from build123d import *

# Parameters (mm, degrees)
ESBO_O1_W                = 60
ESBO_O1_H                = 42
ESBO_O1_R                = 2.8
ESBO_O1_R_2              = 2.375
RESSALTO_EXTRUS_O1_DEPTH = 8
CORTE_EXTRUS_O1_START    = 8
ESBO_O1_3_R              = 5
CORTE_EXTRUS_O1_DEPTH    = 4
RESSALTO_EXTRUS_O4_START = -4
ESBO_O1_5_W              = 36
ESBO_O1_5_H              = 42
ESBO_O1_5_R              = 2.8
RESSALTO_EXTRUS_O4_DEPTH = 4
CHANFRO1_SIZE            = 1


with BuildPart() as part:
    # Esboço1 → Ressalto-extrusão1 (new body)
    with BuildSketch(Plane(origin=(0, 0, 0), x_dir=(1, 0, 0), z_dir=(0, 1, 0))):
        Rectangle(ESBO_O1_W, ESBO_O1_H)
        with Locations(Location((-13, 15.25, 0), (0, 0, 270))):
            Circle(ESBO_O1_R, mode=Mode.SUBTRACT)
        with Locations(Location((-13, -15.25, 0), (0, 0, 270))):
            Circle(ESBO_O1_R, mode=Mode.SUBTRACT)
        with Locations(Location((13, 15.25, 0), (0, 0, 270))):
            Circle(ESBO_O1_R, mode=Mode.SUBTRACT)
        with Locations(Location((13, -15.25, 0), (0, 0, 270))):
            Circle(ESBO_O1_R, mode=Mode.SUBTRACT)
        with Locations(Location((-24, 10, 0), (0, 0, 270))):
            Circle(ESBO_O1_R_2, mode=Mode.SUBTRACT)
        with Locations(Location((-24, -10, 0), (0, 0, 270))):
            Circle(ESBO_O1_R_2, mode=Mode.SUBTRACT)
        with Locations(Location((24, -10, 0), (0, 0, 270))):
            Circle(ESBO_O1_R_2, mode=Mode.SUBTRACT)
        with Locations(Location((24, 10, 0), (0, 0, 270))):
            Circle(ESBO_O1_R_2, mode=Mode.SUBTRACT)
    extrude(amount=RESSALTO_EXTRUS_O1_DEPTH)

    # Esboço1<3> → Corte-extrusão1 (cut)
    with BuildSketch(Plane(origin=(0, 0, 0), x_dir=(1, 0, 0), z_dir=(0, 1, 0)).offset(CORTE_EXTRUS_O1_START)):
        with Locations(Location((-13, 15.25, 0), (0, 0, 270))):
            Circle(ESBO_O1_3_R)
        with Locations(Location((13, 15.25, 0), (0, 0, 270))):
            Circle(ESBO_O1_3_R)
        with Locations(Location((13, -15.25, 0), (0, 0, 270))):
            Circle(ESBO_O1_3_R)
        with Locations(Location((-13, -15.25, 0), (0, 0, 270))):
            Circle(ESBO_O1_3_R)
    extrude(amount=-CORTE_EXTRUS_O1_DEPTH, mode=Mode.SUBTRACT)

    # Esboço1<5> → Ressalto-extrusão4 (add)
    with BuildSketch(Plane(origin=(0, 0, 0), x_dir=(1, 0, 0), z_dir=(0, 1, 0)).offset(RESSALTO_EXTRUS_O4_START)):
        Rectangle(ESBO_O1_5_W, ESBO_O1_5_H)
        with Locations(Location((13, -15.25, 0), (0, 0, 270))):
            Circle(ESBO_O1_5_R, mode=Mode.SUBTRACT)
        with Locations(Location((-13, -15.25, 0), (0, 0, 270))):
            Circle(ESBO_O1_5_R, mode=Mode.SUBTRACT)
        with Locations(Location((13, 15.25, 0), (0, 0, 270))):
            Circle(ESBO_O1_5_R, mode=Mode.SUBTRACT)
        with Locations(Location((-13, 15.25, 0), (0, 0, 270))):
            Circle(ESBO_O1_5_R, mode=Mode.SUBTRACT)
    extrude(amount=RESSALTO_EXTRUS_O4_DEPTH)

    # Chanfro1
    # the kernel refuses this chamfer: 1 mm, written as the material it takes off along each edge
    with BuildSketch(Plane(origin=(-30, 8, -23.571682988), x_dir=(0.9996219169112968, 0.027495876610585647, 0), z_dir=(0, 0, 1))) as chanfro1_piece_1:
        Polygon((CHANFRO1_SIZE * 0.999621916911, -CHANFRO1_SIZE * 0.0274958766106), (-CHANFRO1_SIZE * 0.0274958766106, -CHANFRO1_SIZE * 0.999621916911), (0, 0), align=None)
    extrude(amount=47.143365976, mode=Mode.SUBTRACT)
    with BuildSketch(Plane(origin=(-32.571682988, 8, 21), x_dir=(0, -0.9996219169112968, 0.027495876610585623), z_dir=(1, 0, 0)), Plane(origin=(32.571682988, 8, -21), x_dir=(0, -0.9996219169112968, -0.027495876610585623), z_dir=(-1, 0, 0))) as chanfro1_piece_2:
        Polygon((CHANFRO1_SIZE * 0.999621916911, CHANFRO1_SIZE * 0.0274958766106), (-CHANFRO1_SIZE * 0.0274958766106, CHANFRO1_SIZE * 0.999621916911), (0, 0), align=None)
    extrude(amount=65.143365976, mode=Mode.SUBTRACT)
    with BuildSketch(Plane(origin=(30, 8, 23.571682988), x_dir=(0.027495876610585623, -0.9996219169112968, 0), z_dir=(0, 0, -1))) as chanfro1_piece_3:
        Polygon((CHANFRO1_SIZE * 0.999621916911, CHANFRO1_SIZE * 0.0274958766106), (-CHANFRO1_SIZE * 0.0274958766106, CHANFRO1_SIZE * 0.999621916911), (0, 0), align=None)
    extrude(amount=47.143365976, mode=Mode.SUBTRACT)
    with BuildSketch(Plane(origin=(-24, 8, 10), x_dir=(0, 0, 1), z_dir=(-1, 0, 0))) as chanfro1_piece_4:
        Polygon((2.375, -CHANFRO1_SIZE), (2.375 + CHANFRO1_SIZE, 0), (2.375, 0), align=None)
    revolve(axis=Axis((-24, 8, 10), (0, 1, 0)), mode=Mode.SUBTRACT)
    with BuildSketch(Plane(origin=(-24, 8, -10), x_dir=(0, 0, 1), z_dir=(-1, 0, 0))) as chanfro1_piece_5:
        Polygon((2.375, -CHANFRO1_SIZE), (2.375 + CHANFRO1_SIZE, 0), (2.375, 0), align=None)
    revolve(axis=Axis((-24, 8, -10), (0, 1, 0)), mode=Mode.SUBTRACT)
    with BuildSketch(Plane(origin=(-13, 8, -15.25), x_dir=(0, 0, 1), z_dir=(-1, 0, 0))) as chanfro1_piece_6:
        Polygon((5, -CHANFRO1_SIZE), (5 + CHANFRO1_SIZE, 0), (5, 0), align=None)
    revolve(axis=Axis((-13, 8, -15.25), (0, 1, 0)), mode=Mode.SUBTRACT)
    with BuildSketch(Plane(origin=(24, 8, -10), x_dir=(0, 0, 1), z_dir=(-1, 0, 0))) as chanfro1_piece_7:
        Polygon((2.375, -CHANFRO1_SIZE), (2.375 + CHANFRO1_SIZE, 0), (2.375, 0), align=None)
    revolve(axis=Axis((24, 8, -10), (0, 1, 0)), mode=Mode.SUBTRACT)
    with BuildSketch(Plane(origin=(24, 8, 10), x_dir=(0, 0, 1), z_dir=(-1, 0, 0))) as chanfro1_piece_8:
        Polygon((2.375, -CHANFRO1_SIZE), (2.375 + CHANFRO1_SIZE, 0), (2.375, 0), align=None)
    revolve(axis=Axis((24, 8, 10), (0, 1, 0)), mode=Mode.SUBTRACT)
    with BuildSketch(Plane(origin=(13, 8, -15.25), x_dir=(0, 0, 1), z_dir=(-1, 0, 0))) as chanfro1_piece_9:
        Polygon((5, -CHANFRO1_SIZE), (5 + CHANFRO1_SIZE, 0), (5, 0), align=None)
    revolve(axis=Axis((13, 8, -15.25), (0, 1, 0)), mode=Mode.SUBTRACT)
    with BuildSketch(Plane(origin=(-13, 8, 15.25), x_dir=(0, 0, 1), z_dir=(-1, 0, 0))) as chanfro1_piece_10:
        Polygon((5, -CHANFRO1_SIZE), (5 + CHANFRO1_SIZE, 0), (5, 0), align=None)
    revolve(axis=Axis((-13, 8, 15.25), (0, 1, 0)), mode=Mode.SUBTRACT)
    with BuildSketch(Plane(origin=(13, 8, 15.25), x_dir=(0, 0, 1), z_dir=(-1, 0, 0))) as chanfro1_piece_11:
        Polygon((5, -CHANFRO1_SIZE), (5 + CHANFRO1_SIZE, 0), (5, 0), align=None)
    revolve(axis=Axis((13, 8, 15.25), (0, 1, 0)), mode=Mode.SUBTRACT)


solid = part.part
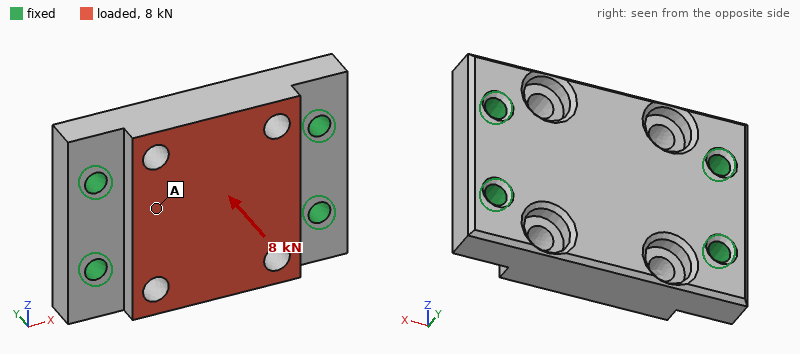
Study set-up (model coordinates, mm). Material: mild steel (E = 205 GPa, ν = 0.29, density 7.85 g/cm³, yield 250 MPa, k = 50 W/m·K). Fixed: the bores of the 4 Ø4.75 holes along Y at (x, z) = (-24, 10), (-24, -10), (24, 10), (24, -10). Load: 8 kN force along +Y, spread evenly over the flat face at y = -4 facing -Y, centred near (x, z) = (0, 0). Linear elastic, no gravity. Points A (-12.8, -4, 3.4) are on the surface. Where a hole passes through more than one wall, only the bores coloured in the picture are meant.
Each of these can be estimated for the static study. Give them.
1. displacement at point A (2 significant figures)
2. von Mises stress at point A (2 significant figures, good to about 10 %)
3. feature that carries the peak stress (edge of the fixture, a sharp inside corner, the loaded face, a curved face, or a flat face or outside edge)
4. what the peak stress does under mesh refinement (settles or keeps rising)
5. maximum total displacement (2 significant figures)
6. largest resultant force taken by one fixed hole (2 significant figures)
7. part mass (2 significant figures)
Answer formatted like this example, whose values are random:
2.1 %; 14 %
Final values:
5.3 µm; 16 MPa; edge of the fixture; keeps rising; 9.4 µm; 2.2 kN; 180 g
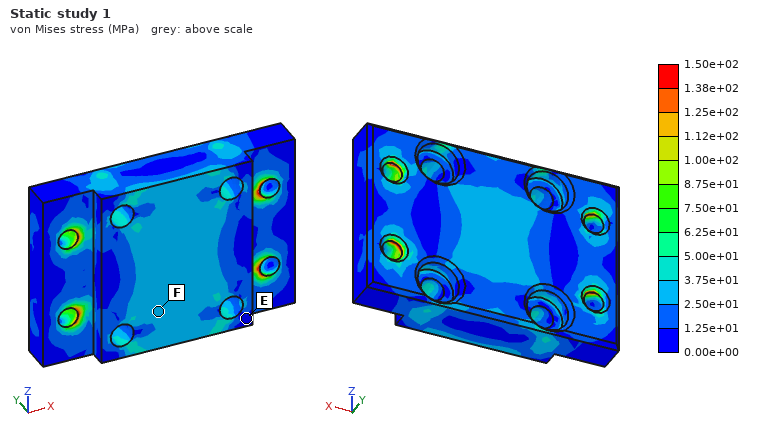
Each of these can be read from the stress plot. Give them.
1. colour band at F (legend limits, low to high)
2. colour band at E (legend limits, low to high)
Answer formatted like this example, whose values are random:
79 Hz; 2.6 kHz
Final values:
2.50e+01 to 3.75e+01 MPa; 0.00e+00 to 1.25e+01 MPa
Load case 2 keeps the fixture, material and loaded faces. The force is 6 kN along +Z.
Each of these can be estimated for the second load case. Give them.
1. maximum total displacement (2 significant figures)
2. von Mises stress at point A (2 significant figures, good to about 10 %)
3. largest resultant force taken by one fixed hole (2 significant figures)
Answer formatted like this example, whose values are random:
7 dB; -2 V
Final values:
7.2 µm; 25 MPa; 2.0 kN
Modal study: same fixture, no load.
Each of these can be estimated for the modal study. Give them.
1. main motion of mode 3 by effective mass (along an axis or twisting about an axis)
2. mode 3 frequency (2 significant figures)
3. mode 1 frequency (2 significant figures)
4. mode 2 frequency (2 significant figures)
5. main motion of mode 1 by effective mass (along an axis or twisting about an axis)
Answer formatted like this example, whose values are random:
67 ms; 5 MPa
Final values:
along Z; 24 kHz; 15 kHz; 16 kHz; along Y
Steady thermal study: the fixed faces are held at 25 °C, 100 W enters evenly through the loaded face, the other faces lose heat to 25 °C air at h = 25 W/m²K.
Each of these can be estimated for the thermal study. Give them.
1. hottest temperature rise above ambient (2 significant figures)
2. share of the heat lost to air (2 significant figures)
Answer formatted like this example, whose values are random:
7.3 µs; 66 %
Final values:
56 K; 4.0 %
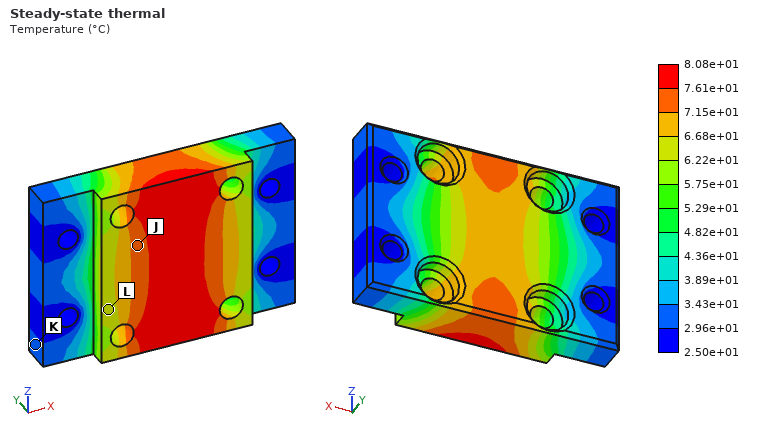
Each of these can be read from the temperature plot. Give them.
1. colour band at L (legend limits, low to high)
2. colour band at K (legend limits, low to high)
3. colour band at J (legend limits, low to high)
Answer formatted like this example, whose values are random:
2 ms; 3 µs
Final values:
6.22e+01 to 6.68e+01 °C; 2.96e+01 to 3.43e+01 °C; 7.15e+01 to 7.61e+01 °C
